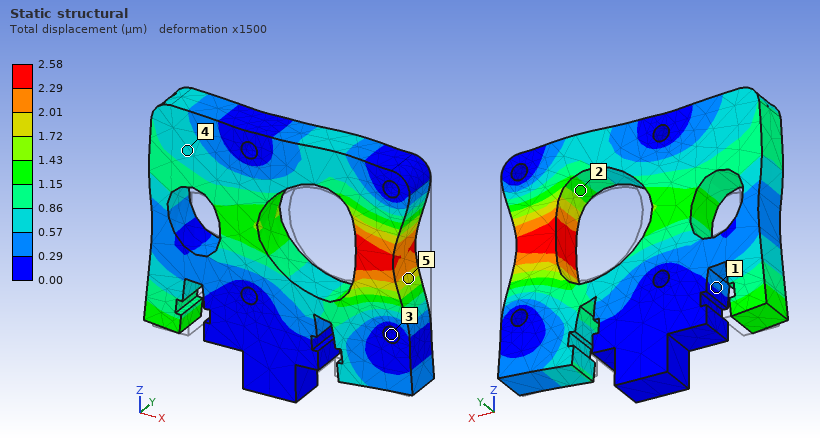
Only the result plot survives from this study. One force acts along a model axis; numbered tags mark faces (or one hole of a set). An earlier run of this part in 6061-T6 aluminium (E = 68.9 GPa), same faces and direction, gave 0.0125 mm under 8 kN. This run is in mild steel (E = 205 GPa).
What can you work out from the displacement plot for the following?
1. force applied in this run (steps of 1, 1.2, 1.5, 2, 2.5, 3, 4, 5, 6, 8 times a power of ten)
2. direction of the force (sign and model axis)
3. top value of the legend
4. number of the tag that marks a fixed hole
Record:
5 kN
-X
2.58 µm
3
